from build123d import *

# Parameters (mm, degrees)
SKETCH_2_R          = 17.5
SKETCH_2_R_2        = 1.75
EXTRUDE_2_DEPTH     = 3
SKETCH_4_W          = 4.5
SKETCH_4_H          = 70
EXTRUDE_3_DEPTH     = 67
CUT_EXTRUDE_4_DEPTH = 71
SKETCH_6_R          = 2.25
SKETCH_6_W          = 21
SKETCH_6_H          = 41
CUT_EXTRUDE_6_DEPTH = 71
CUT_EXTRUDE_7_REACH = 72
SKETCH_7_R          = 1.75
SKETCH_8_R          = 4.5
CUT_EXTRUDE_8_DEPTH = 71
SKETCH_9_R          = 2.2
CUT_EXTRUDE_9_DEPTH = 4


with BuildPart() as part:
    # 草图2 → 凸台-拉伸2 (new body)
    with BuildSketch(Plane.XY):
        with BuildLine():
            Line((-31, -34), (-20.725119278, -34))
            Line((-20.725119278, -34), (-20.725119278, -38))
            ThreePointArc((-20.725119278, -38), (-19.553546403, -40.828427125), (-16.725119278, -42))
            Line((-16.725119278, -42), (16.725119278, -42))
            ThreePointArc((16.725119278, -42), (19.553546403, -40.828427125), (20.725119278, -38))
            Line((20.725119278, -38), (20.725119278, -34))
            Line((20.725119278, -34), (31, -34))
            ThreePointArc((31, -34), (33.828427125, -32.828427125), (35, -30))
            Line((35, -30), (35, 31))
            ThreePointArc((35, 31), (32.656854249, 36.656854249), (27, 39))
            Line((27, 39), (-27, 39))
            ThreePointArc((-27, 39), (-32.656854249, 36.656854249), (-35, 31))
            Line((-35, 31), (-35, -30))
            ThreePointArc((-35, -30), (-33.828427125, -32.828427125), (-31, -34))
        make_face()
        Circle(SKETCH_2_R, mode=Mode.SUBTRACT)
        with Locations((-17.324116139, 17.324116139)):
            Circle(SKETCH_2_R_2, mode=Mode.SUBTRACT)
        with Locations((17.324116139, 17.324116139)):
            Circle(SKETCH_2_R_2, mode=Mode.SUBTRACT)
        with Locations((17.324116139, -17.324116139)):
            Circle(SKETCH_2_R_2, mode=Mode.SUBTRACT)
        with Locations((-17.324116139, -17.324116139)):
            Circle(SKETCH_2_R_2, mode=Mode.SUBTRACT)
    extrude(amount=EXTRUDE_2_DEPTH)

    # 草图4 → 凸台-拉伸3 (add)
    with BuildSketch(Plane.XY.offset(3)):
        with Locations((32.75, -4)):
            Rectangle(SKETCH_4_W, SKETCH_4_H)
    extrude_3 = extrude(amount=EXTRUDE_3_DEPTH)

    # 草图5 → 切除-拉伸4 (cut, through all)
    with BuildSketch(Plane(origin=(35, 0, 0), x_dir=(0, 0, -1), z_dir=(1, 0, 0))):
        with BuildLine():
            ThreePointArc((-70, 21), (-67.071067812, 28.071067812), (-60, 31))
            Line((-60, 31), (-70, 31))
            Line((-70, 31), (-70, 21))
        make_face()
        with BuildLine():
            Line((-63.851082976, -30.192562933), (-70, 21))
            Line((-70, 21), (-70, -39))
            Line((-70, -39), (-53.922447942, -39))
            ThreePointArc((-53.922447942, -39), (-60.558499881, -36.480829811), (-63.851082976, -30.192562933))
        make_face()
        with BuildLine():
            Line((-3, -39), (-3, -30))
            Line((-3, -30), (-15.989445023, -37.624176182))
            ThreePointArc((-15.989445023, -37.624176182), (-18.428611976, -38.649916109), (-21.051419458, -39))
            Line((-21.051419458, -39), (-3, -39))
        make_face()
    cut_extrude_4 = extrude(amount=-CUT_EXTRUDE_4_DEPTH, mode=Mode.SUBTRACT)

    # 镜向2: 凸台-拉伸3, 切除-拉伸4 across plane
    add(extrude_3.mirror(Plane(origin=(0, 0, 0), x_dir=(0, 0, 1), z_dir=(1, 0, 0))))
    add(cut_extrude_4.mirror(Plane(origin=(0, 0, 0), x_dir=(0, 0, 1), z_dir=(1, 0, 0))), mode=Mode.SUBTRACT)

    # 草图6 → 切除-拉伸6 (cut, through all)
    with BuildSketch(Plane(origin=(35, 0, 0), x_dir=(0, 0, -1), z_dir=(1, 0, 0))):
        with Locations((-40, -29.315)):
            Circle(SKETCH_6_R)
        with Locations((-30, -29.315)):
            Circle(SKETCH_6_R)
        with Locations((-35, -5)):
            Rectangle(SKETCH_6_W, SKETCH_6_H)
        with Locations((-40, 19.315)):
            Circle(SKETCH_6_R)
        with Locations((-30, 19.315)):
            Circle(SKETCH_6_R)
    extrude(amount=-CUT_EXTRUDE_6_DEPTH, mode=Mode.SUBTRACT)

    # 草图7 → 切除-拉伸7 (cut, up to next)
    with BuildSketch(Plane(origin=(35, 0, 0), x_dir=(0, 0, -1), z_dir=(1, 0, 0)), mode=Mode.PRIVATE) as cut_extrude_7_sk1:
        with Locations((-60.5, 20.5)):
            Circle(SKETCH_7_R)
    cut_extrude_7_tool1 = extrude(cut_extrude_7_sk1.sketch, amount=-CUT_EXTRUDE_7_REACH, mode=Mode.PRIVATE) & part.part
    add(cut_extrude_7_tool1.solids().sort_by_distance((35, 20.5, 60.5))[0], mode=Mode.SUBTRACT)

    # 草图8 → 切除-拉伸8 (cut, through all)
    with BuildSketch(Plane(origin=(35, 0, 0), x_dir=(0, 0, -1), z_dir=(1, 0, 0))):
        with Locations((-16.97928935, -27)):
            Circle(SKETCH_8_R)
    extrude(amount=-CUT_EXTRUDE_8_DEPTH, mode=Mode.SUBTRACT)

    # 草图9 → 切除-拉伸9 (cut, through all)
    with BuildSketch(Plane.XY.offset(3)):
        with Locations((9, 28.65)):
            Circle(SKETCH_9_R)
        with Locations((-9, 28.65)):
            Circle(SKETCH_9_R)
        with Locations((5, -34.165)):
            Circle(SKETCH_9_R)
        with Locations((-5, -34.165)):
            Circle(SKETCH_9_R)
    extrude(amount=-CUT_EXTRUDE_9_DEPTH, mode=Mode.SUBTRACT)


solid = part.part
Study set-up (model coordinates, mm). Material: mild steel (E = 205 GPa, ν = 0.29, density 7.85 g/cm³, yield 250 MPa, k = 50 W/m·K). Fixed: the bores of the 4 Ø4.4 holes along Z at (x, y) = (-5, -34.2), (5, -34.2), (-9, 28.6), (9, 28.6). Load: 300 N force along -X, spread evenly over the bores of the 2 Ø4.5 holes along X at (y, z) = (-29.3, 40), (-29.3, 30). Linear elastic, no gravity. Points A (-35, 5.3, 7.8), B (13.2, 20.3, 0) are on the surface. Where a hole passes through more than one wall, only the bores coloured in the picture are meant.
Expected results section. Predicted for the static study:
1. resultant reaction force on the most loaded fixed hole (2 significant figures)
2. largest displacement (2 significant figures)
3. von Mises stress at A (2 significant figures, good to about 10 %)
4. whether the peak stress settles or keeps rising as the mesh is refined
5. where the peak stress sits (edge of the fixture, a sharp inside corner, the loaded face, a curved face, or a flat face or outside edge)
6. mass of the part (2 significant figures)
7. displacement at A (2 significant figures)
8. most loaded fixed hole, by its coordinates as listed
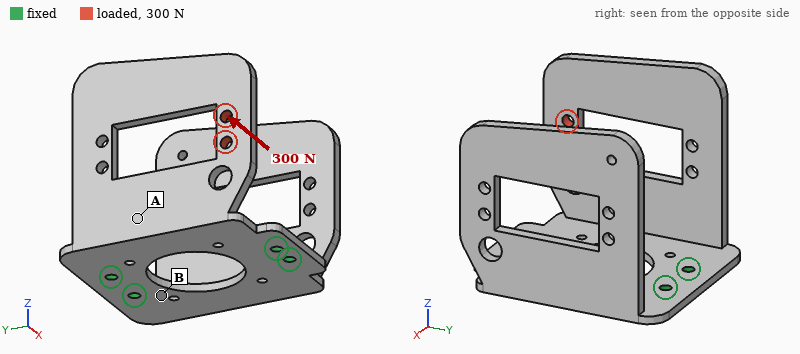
240 N
0.83 mm
35 MPa
keeps rising
edge of the fixture
340 g
0.16 mm
(-5, -34.2)
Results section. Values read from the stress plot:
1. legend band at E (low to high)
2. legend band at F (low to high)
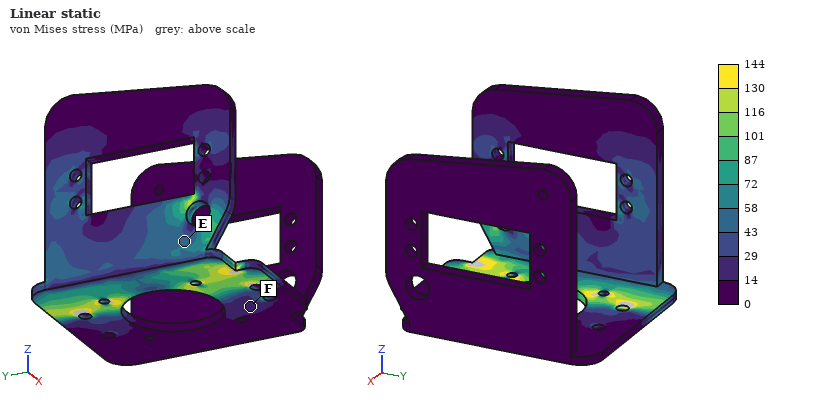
43 to 58 MPa
14 to 29 MPa
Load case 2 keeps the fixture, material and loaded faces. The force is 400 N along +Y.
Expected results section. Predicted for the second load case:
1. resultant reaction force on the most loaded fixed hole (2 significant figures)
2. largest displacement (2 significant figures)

370 N
0.13 mm
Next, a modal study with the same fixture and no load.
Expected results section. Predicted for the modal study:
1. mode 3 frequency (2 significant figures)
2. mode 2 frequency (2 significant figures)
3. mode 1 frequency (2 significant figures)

890 Hz
330 Hz
320 Hz
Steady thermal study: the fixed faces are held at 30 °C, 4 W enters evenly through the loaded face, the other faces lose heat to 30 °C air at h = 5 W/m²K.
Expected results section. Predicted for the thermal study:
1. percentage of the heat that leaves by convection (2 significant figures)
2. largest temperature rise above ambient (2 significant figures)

27 %
40 K
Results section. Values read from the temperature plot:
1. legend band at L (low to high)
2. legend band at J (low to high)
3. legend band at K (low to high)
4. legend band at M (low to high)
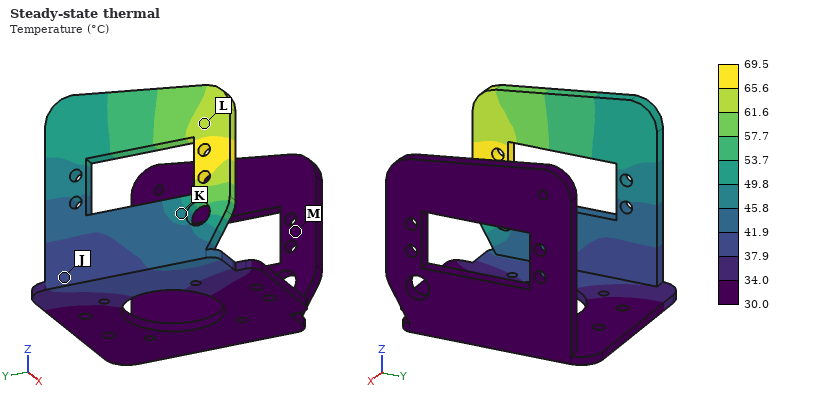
61.6 to 65.6 °C
37.9 to 41.9 °C
45.8 to 49.8 °C
30.0 to 34.0 °C
